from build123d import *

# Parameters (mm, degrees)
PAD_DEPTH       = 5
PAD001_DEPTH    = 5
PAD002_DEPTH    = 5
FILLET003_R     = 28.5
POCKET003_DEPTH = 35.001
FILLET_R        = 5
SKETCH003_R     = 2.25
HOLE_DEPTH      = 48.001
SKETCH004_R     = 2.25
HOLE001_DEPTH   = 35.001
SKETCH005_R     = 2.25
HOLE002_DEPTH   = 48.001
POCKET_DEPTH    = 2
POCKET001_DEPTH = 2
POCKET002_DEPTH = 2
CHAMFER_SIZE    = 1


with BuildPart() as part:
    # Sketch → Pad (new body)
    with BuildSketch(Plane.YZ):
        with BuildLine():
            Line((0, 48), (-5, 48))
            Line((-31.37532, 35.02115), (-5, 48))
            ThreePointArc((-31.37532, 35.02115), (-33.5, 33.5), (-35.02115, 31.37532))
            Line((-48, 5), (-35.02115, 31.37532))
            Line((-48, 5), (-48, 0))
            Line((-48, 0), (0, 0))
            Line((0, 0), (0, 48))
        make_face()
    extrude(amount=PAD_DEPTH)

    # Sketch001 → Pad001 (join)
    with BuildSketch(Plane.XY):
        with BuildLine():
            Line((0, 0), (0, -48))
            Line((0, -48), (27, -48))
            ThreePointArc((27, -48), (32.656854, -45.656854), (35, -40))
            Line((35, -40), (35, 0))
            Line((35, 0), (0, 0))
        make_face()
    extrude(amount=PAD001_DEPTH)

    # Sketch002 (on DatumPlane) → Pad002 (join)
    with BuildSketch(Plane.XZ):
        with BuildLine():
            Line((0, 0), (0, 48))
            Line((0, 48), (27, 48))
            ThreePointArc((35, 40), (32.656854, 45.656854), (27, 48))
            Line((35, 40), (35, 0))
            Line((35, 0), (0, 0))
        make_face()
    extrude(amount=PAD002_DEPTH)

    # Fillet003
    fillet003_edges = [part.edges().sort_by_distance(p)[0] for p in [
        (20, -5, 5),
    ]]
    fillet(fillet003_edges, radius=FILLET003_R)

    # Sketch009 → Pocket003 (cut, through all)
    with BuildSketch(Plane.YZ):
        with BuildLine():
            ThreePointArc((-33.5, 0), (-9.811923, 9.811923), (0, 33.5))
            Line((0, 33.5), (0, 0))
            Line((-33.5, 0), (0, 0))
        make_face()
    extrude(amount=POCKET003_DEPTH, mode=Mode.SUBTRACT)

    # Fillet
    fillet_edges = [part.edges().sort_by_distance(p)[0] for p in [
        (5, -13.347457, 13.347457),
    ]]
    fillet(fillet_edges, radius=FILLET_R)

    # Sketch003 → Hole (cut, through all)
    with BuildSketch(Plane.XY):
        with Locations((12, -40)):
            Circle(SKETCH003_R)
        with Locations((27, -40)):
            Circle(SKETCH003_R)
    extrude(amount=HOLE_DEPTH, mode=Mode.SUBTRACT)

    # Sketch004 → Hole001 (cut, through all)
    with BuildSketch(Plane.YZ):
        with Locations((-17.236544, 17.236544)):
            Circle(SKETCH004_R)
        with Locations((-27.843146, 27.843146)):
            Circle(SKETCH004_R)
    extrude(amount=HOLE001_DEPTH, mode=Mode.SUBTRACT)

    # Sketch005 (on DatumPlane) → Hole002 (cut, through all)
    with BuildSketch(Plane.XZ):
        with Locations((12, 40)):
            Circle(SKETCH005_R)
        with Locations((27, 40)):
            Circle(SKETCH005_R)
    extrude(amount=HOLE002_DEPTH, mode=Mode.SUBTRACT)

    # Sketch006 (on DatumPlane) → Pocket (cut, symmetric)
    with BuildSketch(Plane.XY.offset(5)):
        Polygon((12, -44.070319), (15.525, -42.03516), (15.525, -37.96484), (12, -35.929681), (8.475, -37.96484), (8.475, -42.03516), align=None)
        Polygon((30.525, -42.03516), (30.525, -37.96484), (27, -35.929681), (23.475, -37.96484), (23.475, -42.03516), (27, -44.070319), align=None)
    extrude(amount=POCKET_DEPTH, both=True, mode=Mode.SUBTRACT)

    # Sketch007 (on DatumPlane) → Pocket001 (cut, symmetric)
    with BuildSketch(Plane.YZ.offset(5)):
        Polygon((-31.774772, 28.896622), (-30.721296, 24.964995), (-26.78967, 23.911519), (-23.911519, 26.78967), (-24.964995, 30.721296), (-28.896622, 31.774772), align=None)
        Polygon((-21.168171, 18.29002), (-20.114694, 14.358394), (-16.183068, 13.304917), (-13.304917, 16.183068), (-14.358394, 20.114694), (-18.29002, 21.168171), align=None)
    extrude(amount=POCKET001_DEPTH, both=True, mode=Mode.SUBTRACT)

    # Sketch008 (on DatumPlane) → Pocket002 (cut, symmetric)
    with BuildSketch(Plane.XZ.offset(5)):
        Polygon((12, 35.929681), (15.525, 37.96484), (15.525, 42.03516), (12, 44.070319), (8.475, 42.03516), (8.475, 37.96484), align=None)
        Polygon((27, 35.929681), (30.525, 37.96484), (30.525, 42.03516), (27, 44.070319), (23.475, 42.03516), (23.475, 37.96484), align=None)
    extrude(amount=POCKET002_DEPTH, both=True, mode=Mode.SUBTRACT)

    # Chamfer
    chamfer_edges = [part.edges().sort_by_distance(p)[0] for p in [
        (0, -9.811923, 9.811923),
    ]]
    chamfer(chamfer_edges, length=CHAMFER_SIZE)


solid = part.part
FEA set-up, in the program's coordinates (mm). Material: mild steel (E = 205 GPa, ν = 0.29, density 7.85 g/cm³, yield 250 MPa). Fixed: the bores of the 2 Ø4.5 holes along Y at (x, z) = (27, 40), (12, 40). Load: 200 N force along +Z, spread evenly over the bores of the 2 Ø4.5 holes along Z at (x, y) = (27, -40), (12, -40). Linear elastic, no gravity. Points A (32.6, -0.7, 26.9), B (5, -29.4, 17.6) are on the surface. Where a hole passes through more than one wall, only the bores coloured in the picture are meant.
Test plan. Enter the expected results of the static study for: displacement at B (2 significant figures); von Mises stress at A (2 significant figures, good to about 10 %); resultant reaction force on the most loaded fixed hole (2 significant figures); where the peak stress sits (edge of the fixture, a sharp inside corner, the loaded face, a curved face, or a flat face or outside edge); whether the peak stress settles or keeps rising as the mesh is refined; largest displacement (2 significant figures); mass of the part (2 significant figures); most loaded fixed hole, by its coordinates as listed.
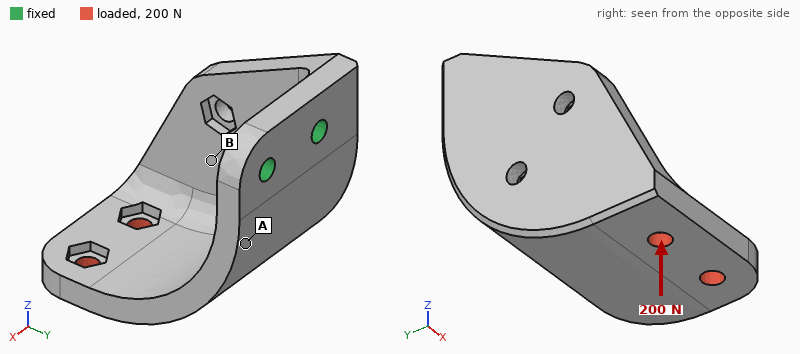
38 µm
19 MPa
160 N
edge of the fixture
keeps rising
78 µm
140 g
(27, 40)
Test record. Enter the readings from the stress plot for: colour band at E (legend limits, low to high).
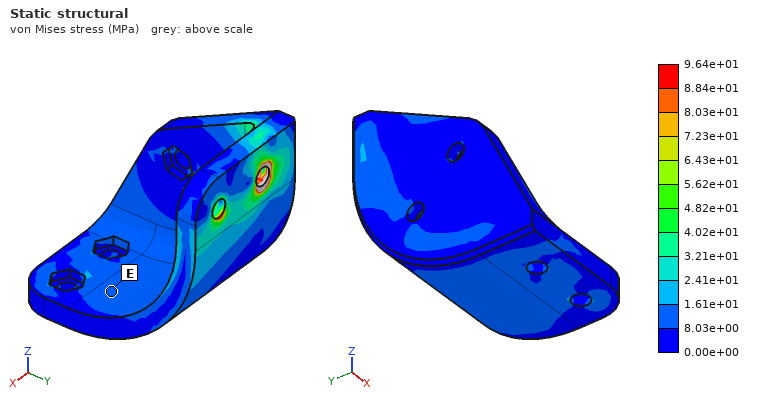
8.03e+00 to 1.61e+01 MPa
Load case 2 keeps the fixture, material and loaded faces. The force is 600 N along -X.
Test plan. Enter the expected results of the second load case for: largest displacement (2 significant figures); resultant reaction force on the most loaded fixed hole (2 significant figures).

0.13 mm
1.9 kN
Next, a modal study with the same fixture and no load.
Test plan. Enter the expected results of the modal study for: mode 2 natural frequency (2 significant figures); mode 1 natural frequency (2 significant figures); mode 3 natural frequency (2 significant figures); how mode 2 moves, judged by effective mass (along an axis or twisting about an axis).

1800 Hz
1100 Hz
5200 Hz
along X
